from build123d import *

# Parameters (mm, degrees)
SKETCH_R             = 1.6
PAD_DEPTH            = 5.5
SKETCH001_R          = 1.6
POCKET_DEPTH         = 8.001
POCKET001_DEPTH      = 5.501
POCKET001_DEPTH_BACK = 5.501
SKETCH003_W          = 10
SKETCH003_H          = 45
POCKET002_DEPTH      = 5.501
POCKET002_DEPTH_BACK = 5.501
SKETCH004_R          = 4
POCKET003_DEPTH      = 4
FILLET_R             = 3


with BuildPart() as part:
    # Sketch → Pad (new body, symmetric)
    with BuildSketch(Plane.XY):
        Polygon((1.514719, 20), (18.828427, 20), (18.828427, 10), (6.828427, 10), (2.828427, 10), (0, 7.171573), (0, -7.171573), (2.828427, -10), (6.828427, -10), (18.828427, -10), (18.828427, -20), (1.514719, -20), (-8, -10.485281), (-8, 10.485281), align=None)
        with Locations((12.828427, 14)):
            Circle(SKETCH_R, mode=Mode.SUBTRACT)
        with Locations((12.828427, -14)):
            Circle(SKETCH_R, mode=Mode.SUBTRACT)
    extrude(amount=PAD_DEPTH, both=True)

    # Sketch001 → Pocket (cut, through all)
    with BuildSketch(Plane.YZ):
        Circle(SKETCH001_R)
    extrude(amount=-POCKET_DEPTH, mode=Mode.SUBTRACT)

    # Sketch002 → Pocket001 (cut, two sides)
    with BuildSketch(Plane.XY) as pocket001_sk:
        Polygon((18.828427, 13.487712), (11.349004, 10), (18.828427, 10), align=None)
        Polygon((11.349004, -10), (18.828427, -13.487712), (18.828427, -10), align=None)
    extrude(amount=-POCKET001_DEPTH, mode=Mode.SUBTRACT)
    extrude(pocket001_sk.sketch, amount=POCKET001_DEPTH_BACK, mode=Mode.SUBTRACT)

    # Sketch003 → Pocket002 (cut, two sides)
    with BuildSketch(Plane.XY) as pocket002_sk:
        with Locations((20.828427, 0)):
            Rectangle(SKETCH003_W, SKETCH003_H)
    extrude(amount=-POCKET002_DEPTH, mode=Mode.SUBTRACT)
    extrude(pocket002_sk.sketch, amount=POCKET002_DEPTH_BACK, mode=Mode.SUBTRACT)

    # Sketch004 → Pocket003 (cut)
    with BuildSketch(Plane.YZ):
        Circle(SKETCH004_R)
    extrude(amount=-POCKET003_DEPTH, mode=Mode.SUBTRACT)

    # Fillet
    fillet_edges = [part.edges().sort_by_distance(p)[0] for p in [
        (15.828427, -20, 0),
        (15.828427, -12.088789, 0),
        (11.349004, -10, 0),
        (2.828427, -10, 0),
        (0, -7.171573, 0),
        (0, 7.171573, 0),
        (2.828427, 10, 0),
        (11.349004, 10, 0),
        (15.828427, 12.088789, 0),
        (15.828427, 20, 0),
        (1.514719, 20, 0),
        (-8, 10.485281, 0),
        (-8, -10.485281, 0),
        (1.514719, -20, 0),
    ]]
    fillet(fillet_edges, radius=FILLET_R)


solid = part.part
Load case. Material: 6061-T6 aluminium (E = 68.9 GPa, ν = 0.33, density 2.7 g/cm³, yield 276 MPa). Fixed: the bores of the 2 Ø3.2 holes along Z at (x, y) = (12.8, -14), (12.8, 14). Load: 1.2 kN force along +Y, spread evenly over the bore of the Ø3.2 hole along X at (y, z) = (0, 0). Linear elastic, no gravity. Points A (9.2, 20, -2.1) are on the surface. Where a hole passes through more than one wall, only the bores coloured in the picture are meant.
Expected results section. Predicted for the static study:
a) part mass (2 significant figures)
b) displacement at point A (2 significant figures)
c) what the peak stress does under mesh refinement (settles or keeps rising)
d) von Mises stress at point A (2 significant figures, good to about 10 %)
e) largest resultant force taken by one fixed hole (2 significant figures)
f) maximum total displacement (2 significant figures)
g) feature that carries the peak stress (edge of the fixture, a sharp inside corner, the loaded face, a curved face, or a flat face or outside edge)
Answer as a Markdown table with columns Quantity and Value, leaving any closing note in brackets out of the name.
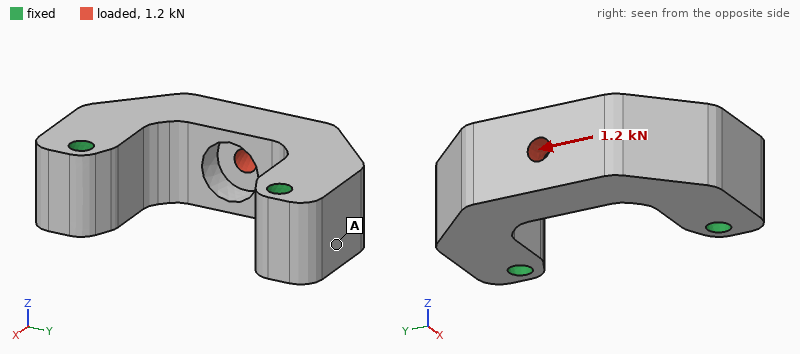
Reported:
| Quantity | Value |
|---|---|
| part mass | 15 g |
| displacement at point A | 5.2 µm |
| what the peak stress does under mesh refinement | keeps rising |
| von Mises stress at point A | 14 MPa |
| largest resultant force taken by one fixed hole | 750 N |
| maximum total displacement | 16 µm |
| feature that carries the peak stress | edge of the fixture |
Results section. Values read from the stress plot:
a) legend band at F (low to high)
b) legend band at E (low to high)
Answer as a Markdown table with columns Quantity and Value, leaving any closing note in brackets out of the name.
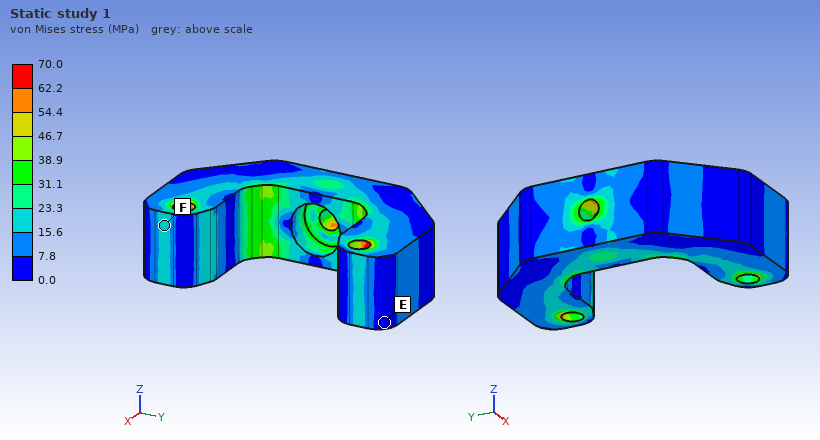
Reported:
| Quantity | Value |
|---|---|
| legend band at F | 15.6 to 23.3 MPa |
| legend band at E | 0.0 to 7.8 MPa |
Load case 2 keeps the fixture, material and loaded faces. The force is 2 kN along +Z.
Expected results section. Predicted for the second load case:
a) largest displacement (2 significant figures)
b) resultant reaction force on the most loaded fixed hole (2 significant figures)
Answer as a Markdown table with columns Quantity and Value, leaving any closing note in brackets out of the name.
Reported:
| Quantity | Value |
|---|---|
| largest displacement | 68 µm |
| resultant reaction force on the most loaded fixed hole | 1.0 kN |
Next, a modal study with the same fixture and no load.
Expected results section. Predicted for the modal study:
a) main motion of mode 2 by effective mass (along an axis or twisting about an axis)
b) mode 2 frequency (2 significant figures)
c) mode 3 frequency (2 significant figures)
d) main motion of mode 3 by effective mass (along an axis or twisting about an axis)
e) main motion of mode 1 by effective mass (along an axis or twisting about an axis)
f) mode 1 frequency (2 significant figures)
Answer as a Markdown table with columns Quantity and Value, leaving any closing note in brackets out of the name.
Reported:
| Quantity | Value |
|---|---|
| main motion of mode 2 by effective mass | along Y |
| mode 2 frequency | 17 kHz |
| mode 3 frequency | 26 kHz |
| main motion of mode 3 by effective mass | twisting about X |
| main motion of mode 1 by effective mass | along Z |
| mode 1 frequency | 14 kHz |
